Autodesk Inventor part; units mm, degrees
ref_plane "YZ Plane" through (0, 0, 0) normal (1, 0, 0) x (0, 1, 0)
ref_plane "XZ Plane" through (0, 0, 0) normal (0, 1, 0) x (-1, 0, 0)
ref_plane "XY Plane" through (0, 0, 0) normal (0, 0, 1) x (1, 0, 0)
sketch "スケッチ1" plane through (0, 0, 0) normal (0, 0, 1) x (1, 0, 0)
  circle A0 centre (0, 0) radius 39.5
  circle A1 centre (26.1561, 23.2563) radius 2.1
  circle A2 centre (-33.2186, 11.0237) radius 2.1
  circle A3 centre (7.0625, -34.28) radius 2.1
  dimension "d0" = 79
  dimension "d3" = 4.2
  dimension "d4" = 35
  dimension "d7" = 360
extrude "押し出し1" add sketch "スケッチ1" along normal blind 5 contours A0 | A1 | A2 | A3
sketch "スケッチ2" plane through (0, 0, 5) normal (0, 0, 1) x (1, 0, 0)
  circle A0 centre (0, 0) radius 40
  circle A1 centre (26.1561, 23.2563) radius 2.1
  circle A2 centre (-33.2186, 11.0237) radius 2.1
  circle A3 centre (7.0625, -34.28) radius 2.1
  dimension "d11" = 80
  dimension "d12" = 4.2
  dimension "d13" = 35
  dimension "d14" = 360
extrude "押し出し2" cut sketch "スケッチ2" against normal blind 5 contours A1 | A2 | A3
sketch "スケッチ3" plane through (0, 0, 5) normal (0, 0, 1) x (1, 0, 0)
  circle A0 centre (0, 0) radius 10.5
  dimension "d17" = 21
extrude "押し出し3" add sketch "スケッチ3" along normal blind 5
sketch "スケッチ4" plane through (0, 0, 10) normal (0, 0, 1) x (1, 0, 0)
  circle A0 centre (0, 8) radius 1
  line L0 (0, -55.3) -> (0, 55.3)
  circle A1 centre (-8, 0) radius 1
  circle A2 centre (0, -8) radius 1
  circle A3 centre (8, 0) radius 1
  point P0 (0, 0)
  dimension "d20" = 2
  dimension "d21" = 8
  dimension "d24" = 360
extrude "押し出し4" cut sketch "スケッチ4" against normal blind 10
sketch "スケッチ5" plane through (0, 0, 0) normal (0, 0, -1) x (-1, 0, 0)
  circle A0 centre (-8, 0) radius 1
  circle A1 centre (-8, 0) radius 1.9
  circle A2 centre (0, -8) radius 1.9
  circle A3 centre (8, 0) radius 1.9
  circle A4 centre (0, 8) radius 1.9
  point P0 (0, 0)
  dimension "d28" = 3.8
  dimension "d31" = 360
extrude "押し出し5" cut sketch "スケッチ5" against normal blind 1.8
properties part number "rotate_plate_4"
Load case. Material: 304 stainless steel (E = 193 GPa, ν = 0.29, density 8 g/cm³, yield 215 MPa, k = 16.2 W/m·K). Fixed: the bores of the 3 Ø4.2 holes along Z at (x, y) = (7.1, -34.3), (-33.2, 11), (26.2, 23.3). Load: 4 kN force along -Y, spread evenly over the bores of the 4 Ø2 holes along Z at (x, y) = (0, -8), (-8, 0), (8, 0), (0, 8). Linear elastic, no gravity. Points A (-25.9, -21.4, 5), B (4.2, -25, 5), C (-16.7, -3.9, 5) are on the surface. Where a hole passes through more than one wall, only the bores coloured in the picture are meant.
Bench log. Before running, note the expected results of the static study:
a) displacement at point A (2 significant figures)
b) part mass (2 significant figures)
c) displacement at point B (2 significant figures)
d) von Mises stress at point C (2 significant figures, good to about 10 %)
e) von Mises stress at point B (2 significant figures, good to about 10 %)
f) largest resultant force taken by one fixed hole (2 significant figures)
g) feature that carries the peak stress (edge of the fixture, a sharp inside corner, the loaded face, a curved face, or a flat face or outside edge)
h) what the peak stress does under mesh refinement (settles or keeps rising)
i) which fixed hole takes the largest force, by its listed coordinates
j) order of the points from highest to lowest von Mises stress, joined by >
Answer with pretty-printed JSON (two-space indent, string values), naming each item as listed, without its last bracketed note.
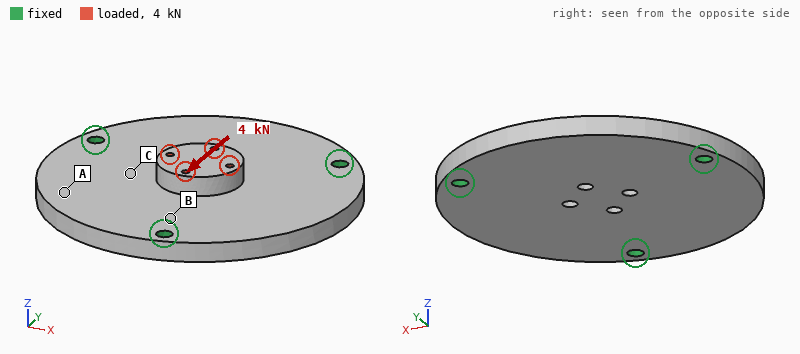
{
  "displacement at point A": "4.6 µm",
  "part mass": "210 g",
  "displacement at point B": "2.0 µm",
  "von Mises stress at point C": "15 MPa",
  "von Mises stress at point B": "24 MPa",
  "largest resultant force taken by one fixed hole": "1.5 kN",
  "feature that carries the peak stress": "edge of the fixture",
  "what the peak stress does under mesh refinement": "keeps rising",
  "which fixed hole takes the largest force, by its listed coordinates": "(7.1, -34.3)",
  "order of the points from highest to lowest von Mises stress, joined by >": "B > C > A"
}
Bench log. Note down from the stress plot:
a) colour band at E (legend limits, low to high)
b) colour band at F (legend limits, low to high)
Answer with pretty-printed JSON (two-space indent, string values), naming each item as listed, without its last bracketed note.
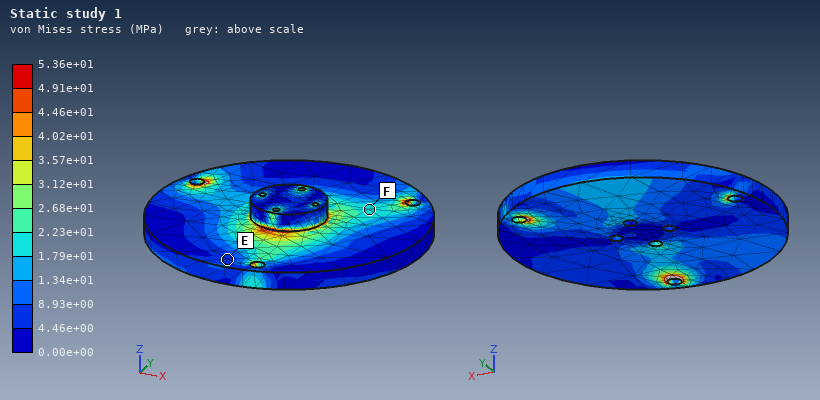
{
  "colour band at E": "4.46e+00 to 8.93e+00 MPa",
  "colour band at F": "1.79e+01 to 2.23e+01 MPa"
}
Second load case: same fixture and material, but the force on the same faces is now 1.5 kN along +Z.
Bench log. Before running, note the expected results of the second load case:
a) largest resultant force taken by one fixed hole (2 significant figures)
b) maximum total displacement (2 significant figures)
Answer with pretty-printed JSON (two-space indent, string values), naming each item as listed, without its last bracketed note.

{
  "largest resultant force taken by one fixed hole": "510 N",
  "maximum total displacement": "17 µm"
}
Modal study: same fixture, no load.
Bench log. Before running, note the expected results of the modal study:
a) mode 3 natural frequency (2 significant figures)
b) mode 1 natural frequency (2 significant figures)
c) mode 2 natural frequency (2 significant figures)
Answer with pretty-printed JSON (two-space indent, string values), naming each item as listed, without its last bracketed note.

{
  "mode 3 natural frequency": "5000 Hz",
  "mode 1 natural frequency": "5000 Hz",
  "mode 2 natural frequency": "5000 Hz"
}
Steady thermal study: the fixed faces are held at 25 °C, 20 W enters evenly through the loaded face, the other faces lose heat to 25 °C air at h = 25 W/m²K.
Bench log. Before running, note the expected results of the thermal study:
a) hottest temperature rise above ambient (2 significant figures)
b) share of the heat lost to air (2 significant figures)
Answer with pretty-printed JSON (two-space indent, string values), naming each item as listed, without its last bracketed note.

{
  "hottest temperature rise above ambient": "79 K",
  "share of the heat lost to air": "41 %"
}
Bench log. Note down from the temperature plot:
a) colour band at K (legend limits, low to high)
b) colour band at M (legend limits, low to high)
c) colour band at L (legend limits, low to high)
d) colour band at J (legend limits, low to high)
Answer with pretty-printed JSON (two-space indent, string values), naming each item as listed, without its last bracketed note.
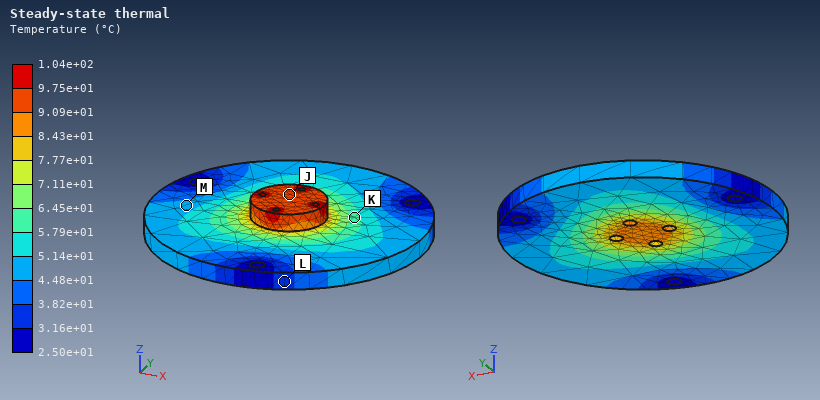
{
  "colour band at K": "5.79e+01 to 6.45e+01 °C",
  "colour band at M": "4.48e+01 to 5.14e+01 °C",
  "colour band at L": "3.16e+01 to 3.82e+01 °C",
  "colour band at J": "9.09e+01 to 9.75e+01 °C"
}
